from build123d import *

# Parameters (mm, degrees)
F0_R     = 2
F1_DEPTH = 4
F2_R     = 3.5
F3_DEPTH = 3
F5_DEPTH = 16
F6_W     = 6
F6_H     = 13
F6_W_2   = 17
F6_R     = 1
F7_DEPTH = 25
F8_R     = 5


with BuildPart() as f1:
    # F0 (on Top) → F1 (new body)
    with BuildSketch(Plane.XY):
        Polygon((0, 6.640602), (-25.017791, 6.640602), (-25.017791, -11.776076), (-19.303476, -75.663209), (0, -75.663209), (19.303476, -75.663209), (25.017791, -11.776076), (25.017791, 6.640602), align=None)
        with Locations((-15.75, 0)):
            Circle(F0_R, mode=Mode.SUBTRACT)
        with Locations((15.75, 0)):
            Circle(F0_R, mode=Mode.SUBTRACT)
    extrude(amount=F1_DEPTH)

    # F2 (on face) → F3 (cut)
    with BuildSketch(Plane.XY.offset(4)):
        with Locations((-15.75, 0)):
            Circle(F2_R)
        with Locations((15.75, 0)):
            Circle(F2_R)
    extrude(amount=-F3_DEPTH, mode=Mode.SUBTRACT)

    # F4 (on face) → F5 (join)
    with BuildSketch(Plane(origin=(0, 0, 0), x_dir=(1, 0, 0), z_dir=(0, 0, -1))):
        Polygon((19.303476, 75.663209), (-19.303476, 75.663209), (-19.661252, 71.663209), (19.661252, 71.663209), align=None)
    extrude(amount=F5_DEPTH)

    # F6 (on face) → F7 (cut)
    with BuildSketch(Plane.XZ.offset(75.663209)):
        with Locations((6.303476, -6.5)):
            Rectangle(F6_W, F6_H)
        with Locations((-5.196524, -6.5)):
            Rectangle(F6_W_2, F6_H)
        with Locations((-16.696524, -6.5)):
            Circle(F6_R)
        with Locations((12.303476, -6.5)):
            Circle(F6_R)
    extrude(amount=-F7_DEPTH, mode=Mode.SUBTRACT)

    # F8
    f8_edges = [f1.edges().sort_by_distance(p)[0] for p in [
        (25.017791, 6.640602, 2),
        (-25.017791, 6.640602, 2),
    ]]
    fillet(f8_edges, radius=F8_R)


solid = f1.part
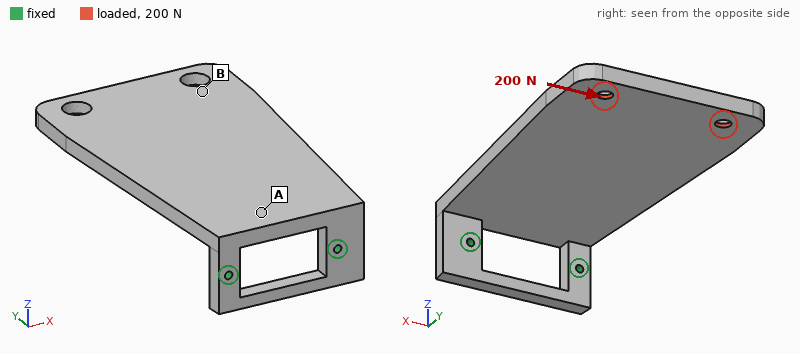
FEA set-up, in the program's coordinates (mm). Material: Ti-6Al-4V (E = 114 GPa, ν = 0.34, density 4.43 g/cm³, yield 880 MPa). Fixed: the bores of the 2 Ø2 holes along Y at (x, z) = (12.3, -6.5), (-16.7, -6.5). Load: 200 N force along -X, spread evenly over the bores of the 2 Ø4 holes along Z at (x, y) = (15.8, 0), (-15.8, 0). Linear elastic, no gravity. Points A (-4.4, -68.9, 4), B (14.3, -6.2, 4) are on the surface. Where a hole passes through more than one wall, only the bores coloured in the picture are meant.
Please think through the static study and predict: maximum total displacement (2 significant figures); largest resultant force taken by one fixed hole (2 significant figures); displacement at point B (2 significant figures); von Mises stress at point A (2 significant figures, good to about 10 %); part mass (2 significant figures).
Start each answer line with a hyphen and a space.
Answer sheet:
- 0.10 mm
- 480 N
- 0.078 mm
- 21 MPa
- 71 g
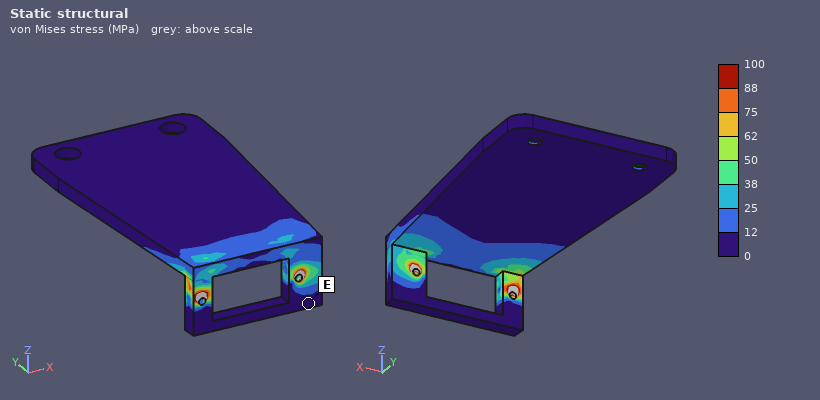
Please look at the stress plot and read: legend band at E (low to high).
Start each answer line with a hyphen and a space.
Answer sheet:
- 0 to 12 MPa
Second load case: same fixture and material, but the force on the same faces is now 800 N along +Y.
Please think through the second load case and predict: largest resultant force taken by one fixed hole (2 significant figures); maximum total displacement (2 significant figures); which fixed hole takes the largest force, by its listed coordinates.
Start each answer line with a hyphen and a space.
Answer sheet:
- 450 N
- 57 µm
- (12.3, -6.5)
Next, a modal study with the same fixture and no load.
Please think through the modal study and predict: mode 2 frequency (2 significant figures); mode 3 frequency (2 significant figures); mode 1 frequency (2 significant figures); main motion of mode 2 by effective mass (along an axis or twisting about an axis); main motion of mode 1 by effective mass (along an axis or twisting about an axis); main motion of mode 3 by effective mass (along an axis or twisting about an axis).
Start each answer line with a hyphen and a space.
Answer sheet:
- 1400 Hz
- 1800 Hz
- 330 Hz
- along X
- along Z
- along X
